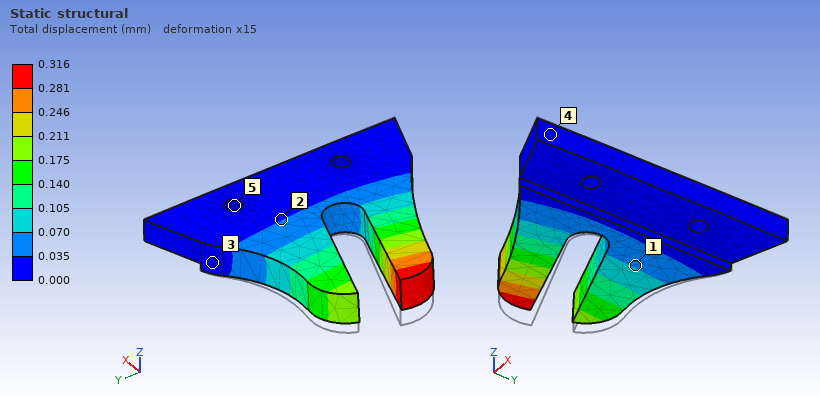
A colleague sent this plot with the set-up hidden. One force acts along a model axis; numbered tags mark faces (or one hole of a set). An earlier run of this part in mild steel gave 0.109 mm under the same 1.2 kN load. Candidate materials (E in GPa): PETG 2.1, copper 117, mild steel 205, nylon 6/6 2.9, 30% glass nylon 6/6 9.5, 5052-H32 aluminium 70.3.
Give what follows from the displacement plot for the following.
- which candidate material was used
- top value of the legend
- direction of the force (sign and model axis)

5052-H32 aluminium
0.316 mm
+Z
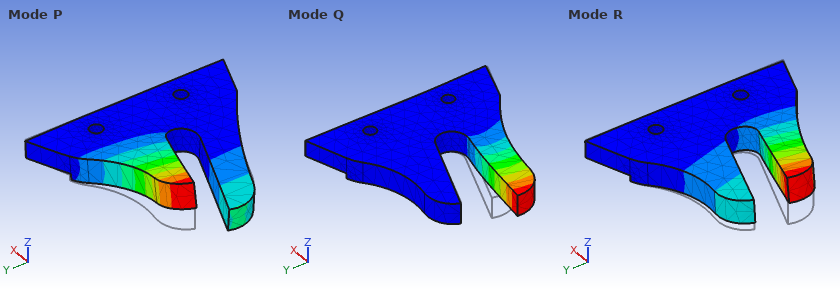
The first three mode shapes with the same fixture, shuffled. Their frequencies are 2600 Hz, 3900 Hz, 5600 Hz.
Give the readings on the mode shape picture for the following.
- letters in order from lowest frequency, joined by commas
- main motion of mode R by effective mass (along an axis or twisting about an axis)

R, P, Q
along Z
